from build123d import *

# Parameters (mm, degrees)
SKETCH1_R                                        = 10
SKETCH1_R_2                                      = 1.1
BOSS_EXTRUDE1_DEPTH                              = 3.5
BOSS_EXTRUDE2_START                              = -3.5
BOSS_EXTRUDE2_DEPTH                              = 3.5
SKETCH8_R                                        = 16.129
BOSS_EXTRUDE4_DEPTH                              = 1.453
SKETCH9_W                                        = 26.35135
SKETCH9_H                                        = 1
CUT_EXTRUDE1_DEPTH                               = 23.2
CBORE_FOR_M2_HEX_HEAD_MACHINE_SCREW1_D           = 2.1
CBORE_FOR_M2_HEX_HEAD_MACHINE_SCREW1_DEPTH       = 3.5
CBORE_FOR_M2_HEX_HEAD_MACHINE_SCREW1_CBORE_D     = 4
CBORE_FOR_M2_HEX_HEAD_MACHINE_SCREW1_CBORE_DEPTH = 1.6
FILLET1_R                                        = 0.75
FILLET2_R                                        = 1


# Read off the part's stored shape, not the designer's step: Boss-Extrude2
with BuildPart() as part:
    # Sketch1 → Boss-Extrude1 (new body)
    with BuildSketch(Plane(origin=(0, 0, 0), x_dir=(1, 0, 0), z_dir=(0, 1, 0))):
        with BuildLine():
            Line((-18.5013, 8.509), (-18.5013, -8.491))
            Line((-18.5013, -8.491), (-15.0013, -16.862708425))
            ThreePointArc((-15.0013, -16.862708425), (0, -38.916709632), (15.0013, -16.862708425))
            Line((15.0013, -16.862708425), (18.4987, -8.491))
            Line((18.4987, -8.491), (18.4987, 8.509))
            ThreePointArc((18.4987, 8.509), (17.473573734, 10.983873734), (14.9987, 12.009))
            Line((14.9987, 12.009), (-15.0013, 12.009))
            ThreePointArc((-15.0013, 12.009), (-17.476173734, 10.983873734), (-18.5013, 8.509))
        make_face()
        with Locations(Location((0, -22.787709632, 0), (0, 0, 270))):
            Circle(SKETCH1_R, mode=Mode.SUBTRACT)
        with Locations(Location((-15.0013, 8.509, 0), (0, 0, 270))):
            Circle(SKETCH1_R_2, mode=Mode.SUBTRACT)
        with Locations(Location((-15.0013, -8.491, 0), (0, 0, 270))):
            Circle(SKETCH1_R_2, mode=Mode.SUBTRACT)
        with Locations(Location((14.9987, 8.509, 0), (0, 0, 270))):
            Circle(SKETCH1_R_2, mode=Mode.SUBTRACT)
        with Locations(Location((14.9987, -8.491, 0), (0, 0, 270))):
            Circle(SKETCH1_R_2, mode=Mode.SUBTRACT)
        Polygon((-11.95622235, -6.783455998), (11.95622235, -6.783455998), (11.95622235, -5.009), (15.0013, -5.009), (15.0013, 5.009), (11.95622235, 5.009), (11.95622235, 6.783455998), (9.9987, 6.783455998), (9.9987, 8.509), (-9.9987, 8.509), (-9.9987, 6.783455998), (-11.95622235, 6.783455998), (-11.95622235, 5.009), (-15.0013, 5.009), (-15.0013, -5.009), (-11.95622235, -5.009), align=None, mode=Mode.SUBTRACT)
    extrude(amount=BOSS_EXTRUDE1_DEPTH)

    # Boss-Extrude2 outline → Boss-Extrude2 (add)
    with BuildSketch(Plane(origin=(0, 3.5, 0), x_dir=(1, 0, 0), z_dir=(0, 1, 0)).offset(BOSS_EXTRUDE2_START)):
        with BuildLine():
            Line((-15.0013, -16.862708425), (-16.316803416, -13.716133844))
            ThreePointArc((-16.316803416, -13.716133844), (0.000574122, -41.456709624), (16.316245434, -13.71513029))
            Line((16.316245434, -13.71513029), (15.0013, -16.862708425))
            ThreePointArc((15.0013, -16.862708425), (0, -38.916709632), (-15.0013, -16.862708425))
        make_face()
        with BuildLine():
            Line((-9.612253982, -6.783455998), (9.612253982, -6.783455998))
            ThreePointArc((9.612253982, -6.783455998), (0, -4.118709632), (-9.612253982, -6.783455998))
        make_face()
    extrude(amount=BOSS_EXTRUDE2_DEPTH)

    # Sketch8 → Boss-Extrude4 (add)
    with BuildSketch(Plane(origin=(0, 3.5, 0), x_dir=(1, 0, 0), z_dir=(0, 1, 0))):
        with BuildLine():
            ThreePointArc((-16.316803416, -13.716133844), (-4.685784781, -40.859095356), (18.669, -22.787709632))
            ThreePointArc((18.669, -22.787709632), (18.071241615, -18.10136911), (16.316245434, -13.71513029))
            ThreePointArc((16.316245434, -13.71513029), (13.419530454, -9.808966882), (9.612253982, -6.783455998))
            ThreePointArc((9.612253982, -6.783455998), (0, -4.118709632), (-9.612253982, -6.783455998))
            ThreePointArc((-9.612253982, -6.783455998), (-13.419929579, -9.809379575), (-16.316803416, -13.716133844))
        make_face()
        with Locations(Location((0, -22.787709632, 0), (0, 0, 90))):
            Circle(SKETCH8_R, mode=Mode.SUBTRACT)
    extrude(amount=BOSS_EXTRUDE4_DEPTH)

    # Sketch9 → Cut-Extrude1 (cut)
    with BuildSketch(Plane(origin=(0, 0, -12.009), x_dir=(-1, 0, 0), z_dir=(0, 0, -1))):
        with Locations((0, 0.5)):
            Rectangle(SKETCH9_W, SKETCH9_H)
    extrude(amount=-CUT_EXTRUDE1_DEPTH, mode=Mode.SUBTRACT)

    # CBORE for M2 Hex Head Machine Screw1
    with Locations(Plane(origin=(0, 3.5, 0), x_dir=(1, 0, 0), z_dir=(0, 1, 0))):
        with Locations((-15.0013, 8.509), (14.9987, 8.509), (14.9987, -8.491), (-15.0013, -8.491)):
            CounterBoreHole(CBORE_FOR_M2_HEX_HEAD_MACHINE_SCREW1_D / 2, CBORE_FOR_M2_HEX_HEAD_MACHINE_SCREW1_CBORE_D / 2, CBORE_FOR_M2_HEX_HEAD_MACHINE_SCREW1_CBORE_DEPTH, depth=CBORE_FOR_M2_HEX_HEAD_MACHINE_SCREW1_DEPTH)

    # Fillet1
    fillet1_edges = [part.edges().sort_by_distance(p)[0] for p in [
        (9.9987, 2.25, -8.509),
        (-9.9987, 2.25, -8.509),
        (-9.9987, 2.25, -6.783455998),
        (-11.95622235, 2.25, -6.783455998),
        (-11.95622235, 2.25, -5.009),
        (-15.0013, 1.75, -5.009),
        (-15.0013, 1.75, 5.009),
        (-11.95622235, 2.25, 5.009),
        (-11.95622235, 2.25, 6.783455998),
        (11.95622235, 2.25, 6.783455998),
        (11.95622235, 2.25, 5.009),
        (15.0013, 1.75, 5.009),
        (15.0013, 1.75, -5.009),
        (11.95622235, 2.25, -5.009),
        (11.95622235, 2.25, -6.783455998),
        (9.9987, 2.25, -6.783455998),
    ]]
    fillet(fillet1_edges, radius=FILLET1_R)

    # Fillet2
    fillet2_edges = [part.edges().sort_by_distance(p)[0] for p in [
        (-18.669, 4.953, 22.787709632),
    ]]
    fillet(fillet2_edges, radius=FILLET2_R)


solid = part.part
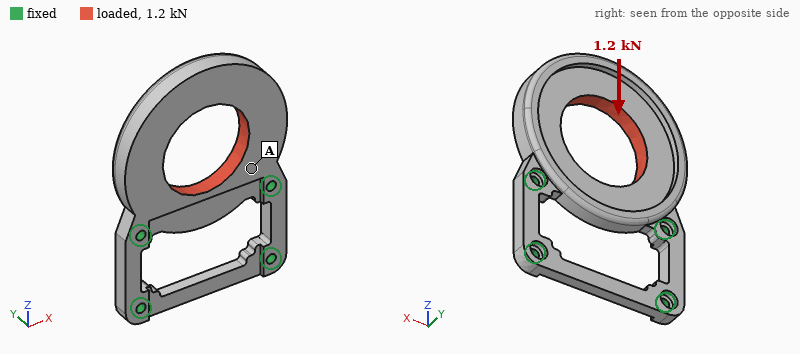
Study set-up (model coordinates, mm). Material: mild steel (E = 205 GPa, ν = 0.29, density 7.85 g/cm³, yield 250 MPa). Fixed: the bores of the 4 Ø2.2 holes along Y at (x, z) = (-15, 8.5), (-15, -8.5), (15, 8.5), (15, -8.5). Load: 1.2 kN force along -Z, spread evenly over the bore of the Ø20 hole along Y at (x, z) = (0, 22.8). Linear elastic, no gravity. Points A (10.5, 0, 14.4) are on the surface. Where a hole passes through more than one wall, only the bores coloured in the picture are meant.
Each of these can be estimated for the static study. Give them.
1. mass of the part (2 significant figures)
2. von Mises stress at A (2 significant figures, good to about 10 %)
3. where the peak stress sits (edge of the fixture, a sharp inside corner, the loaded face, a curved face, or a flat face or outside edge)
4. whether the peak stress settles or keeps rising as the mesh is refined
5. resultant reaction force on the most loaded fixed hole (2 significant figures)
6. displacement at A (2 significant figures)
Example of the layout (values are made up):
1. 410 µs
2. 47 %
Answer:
1. 31 g
2. 11 MPa
3. edge of the fixture
4. keeps rising
5. 590 N
6. 2.1 µm
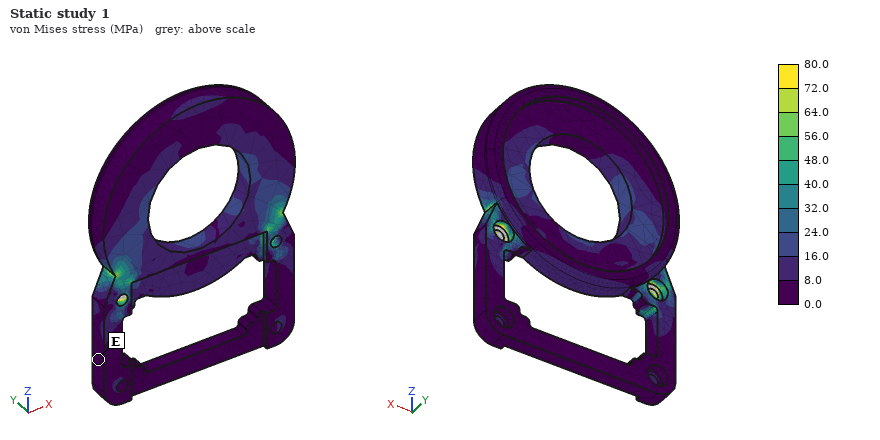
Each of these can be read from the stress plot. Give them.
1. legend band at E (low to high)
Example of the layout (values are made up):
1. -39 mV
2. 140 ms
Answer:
1. 0.0 to 8.0 MPa
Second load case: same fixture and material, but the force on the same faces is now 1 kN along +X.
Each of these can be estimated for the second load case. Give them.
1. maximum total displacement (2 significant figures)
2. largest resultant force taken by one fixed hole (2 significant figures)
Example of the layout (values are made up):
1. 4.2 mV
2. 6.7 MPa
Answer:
1. 13 µm
2. 630 N
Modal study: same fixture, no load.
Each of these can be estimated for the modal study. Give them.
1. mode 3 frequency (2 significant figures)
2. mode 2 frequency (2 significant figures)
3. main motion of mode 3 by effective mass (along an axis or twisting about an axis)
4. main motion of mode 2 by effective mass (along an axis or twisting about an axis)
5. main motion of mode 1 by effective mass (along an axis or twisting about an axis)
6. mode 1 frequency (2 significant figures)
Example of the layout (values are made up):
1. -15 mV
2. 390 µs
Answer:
1. 9700 Hz
2. 6000 Hz
3. along X
4. twisting about Z
5. along Y
6. 1900 Hz
